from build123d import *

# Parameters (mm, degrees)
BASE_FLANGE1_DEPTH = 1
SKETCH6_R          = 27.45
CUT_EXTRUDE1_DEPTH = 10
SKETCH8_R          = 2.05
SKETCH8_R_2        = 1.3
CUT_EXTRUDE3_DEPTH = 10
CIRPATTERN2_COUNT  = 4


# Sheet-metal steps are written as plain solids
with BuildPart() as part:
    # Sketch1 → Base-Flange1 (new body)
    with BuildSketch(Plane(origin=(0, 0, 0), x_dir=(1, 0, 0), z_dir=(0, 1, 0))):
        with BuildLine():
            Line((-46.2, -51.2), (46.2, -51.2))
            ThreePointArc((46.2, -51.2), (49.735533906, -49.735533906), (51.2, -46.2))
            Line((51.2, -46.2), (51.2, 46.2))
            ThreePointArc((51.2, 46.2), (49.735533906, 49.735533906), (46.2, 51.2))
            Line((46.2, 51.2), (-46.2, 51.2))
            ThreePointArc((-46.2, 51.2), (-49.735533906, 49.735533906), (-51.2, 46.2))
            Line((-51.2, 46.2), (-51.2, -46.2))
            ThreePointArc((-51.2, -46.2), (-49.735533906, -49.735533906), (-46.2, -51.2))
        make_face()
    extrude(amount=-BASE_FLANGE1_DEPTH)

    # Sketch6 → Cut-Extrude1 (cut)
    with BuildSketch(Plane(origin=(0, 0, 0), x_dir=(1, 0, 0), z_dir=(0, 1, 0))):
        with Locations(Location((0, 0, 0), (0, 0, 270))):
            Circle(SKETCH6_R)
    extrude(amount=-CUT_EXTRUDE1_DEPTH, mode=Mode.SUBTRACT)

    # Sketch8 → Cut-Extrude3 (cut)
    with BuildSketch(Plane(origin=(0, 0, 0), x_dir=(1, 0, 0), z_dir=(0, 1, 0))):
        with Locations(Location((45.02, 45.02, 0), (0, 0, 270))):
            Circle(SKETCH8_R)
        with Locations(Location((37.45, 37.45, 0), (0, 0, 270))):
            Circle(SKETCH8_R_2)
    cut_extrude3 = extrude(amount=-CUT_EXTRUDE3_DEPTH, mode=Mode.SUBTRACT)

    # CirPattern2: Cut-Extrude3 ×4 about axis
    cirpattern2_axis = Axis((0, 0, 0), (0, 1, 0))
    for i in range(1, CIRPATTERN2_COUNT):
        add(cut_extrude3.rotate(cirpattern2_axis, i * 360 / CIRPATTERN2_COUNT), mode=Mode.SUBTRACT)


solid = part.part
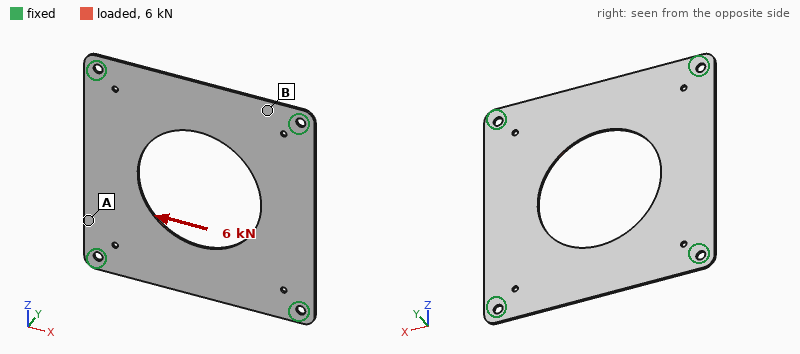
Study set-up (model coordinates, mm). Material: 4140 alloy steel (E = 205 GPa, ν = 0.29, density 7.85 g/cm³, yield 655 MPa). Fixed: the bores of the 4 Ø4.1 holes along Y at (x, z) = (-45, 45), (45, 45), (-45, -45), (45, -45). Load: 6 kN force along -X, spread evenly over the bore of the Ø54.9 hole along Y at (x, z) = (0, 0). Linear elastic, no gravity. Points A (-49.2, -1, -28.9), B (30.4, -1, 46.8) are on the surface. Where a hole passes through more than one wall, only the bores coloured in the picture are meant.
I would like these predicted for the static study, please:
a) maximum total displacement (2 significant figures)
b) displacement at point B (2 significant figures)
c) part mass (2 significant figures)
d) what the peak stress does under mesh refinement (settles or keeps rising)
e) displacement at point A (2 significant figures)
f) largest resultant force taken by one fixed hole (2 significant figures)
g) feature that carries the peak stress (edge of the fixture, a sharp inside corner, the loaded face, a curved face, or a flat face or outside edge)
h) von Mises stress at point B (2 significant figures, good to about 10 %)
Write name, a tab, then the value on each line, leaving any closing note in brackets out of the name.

maximum total displacement	29 µm
displacement at point B	6.4 µm
part mass	63 g
what the peak stress does under mesh refinement	keeps rising
displacement at point A	15 µm
largest resultant force taken by one fixed hole	1.6 kN
feature that carries the peak stress	edge of the fixture
von Mises stress at point B	74 MPa
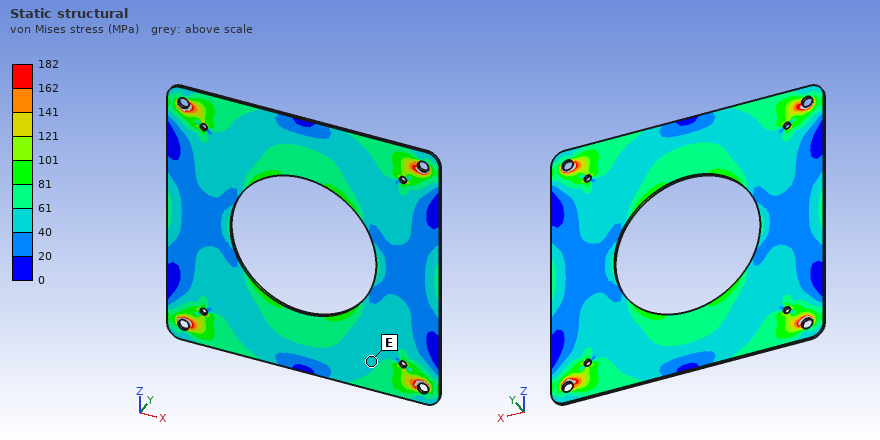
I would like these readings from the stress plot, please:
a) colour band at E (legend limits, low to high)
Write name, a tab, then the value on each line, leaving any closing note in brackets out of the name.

colour band at E	40 to 61 MPa
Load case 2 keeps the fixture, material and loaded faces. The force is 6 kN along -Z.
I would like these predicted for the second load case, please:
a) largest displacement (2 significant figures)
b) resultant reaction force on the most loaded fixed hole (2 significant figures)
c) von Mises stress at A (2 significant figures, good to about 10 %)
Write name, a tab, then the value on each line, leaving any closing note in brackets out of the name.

largest displacement	29 µm
resultant reaction force on the most loaded fixed hole	1.6 kN
von Mises stress at A	74 MPa
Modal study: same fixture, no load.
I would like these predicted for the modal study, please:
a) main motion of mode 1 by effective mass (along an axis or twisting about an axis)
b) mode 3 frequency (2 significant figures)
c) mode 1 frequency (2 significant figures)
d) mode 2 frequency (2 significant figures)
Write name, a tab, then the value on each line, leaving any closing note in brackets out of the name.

main motion of mode 1 by effective mass	along Y
mode 3 frequency	700 Hz
mode 1 frequency	510 Hz
mode 2 frequency	700 Hz
